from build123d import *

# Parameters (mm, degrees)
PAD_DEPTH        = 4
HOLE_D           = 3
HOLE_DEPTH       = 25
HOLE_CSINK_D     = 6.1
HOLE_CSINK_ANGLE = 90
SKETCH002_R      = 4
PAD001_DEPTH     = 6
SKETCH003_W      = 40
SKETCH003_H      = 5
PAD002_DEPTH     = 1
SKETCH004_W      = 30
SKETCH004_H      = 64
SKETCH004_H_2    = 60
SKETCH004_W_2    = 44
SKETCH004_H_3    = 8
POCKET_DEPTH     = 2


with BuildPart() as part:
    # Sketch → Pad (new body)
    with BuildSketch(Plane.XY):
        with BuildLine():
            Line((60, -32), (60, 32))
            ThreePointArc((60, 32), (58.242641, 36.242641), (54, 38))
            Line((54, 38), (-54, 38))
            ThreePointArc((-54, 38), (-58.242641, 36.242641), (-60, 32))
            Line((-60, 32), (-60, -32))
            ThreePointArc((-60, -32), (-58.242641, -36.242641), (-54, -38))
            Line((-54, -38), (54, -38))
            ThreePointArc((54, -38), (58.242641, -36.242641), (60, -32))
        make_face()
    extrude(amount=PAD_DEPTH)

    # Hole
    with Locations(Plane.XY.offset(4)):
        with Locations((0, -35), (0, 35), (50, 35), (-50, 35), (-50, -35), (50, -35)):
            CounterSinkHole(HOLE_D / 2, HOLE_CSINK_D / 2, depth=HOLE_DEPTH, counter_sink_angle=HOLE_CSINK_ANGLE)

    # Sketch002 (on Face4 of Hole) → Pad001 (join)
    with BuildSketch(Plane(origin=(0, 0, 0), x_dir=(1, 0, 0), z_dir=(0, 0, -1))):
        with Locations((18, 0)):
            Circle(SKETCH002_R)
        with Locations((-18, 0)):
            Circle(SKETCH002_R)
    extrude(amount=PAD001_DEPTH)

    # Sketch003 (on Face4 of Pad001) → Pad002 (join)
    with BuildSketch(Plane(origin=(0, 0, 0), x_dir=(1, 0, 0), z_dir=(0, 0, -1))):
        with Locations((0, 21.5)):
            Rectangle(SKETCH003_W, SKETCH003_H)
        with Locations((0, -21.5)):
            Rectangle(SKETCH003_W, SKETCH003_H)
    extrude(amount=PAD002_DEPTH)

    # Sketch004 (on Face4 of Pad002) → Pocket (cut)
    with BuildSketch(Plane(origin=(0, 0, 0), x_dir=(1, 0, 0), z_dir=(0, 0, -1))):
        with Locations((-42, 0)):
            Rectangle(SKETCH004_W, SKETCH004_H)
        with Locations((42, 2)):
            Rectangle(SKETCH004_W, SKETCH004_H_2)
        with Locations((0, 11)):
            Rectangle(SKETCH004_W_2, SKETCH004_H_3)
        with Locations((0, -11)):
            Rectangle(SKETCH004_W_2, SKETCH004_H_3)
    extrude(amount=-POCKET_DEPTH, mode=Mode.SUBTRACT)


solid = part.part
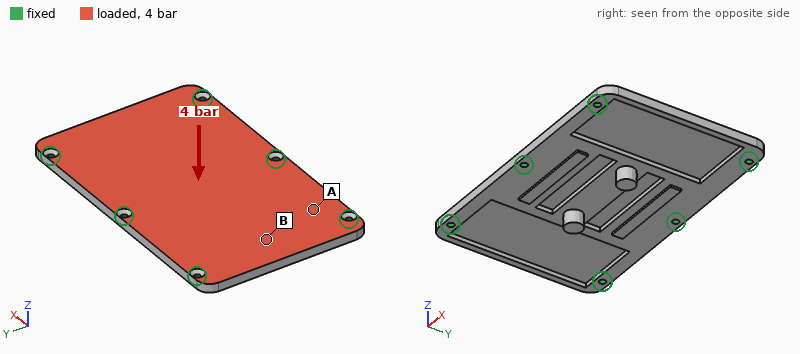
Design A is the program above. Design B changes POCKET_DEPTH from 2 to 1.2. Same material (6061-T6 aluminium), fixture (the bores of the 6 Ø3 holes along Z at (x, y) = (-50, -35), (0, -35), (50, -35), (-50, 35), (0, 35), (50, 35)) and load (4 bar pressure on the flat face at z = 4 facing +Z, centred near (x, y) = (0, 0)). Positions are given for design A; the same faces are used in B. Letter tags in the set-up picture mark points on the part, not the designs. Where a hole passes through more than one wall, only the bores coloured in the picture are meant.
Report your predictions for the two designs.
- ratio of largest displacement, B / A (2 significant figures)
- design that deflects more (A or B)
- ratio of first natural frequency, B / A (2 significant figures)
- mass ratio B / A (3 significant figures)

0.72
A
1.0
1.13
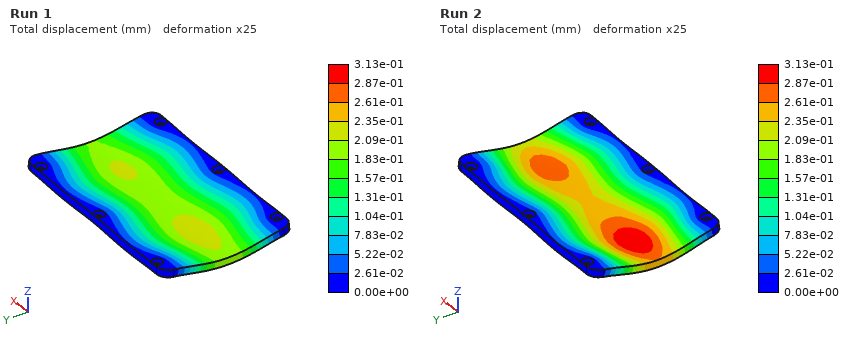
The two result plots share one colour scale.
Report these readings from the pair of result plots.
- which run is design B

Run 1
